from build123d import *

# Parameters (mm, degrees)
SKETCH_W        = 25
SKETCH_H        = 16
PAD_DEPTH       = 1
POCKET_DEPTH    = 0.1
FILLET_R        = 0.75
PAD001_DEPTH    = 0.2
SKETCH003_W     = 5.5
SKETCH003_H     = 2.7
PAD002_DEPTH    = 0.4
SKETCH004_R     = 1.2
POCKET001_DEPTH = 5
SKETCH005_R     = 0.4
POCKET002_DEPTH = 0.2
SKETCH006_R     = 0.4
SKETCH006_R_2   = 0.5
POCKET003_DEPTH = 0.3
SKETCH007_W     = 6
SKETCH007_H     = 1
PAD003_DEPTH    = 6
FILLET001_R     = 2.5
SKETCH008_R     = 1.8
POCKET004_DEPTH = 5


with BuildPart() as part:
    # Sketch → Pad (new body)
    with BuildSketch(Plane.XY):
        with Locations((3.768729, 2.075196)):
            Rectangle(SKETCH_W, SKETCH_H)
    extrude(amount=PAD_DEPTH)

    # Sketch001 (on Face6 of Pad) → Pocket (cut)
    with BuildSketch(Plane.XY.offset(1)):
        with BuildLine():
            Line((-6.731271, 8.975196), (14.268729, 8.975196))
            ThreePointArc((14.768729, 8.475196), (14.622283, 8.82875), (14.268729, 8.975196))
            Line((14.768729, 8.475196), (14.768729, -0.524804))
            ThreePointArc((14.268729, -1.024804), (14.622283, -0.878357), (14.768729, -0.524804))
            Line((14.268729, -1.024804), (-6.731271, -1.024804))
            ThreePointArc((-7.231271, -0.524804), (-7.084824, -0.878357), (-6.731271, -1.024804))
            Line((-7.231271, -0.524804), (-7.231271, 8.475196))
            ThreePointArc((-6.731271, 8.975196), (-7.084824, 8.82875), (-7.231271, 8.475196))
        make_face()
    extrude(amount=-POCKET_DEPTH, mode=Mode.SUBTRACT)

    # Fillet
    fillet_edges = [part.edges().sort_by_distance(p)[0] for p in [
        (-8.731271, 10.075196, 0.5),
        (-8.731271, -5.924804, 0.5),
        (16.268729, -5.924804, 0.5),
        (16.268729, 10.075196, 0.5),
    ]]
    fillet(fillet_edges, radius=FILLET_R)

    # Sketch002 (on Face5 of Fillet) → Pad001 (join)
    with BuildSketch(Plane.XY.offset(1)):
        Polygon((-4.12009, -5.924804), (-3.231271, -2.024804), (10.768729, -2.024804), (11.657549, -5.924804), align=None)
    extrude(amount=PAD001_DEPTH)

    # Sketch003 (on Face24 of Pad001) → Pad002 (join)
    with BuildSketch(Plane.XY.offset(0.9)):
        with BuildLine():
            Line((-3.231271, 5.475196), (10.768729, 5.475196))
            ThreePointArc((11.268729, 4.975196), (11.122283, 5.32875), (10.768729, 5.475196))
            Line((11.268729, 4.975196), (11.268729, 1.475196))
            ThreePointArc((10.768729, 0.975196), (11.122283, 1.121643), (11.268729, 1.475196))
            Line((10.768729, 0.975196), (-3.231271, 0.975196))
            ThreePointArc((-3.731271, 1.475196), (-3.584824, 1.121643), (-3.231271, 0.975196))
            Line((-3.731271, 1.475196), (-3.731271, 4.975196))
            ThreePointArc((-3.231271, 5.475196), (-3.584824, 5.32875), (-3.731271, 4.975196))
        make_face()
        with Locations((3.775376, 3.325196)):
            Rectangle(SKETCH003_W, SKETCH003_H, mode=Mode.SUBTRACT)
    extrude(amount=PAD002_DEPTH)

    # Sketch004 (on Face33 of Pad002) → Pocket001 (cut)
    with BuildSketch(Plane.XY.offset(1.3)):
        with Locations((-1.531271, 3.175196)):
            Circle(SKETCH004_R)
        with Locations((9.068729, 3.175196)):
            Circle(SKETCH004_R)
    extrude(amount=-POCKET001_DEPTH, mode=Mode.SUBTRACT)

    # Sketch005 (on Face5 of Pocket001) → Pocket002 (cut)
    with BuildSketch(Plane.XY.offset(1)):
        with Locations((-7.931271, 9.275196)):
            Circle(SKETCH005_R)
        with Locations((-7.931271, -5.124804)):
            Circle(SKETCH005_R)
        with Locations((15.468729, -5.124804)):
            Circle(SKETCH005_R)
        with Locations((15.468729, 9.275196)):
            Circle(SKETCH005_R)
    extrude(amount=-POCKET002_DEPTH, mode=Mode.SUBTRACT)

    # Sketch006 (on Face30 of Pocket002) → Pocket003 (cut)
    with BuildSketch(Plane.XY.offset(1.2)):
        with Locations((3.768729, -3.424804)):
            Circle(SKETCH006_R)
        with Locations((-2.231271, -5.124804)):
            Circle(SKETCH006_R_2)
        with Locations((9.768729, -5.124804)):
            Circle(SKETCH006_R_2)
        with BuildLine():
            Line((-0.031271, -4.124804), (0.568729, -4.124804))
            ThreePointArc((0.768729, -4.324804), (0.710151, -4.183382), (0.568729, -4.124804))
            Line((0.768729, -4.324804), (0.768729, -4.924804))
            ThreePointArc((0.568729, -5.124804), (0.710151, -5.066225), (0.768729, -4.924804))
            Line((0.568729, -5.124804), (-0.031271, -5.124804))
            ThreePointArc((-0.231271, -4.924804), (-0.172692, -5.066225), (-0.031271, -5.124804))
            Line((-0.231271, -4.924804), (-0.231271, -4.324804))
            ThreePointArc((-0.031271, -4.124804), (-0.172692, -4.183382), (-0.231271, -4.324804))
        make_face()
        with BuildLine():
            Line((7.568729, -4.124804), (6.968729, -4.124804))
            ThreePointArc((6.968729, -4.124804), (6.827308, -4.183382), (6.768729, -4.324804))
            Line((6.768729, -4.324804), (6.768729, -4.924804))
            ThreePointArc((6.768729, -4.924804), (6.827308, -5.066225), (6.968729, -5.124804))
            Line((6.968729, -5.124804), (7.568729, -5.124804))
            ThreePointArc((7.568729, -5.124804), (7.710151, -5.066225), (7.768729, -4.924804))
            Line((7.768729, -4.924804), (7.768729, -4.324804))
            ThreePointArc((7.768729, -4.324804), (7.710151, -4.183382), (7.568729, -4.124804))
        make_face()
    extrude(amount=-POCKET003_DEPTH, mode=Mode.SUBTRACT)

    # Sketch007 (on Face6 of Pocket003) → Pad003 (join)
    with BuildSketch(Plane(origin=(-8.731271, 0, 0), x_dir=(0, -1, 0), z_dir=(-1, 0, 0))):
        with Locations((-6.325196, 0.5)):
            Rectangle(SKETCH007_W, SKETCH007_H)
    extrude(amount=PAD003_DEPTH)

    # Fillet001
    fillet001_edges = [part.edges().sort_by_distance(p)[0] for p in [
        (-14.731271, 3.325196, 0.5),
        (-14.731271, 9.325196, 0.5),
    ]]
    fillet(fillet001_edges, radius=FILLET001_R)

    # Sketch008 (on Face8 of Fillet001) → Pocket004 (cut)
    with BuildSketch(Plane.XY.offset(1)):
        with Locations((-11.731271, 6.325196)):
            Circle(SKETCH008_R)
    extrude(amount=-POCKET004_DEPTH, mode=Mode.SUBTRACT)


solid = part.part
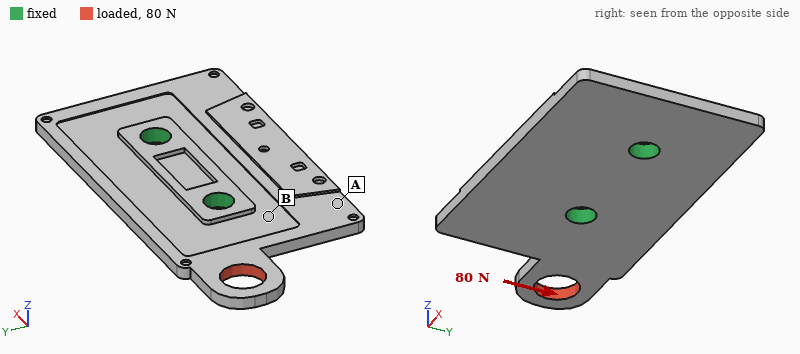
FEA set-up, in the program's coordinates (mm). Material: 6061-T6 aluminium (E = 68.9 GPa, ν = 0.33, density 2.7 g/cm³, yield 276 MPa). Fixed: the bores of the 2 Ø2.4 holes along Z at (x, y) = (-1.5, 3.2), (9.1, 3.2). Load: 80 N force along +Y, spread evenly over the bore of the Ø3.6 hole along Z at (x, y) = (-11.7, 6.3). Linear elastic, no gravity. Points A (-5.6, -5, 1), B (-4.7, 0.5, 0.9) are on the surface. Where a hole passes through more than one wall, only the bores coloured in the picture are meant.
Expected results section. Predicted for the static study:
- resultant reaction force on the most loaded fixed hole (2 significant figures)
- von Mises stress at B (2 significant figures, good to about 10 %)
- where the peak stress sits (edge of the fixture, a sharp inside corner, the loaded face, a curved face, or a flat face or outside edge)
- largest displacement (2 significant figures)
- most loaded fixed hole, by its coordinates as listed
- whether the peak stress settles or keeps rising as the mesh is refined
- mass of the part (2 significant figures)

130 N
21 MPa
a sharp inside corner
24 µm
(-1.5, 3.2)
keeps rising
1.1 g
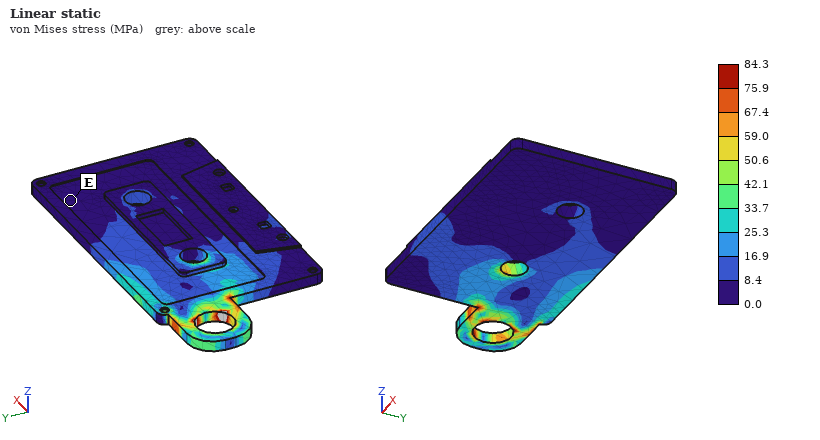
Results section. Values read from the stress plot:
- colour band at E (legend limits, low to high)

0.0 to 8.4 MPa
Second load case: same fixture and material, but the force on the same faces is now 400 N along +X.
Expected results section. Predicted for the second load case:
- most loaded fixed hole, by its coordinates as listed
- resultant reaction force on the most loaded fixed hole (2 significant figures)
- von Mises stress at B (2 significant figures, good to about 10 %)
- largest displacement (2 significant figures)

(-1.5, 3.2)
330 N
18 MPa
28 µm
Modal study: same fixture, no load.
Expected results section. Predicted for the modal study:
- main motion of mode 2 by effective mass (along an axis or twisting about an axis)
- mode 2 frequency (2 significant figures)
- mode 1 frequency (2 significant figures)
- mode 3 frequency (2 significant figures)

along Z
10 kHz
7500 Hz
12 kHz
